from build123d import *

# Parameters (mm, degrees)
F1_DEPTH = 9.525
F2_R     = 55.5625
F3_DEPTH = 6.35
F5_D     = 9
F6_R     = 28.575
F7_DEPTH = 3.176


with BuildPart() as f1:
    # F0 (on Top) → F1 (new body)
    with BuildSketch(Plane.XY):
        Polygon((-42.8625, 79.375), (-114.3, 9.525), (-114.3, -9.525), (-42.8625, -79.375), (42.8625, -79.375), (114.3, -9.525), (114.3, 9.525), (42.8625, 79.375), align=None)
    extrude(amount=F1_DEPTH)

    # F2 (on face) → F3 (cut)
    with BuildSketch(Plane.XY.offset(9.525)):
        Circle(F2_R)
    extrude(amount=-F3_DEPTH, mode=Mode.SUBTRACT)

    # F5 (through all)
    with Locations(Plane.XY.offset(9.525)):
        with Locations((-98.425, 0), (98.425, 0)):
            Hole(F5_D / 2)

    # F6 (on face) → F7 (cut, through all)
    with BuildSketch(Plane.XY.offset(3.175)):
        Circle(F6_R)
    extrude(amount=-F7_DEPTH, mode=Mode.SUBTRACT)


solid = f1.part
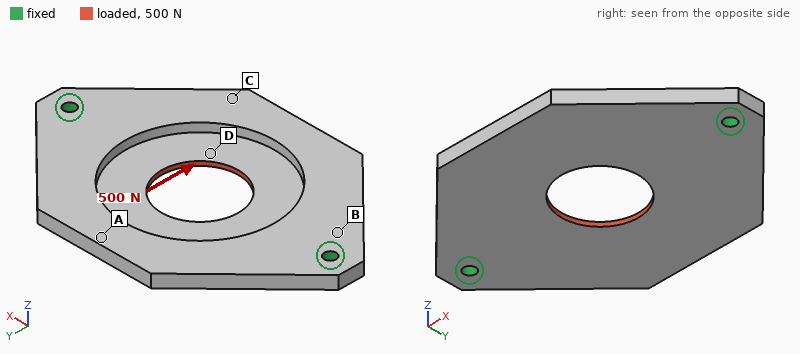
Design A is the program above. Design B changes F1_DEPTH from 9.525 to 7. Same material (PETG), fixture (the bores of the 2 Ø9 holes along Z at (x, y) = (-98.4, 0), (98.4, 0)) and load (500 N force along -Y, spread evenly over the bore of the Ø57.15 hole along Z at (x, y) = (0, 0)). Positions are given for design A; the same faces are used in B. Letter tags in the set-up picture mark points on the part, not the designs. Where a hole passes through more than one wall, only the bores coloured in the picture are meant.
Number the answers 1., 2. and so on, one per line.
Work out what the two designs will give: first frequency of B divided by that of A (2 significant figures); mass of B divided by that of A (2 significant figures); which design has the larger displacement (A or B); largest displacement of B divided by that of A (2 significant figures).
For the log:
1. 0.75
2. 0.77
3. B
4. 1.4
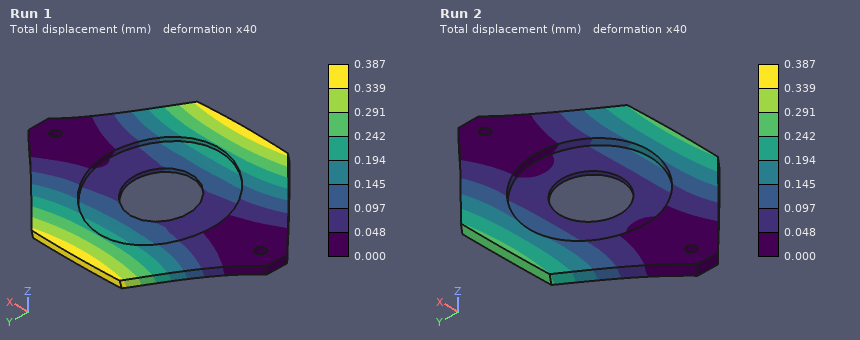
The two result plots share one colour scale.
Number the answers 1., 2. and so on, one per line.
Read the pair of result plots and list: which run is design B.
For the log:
1. Run 1
